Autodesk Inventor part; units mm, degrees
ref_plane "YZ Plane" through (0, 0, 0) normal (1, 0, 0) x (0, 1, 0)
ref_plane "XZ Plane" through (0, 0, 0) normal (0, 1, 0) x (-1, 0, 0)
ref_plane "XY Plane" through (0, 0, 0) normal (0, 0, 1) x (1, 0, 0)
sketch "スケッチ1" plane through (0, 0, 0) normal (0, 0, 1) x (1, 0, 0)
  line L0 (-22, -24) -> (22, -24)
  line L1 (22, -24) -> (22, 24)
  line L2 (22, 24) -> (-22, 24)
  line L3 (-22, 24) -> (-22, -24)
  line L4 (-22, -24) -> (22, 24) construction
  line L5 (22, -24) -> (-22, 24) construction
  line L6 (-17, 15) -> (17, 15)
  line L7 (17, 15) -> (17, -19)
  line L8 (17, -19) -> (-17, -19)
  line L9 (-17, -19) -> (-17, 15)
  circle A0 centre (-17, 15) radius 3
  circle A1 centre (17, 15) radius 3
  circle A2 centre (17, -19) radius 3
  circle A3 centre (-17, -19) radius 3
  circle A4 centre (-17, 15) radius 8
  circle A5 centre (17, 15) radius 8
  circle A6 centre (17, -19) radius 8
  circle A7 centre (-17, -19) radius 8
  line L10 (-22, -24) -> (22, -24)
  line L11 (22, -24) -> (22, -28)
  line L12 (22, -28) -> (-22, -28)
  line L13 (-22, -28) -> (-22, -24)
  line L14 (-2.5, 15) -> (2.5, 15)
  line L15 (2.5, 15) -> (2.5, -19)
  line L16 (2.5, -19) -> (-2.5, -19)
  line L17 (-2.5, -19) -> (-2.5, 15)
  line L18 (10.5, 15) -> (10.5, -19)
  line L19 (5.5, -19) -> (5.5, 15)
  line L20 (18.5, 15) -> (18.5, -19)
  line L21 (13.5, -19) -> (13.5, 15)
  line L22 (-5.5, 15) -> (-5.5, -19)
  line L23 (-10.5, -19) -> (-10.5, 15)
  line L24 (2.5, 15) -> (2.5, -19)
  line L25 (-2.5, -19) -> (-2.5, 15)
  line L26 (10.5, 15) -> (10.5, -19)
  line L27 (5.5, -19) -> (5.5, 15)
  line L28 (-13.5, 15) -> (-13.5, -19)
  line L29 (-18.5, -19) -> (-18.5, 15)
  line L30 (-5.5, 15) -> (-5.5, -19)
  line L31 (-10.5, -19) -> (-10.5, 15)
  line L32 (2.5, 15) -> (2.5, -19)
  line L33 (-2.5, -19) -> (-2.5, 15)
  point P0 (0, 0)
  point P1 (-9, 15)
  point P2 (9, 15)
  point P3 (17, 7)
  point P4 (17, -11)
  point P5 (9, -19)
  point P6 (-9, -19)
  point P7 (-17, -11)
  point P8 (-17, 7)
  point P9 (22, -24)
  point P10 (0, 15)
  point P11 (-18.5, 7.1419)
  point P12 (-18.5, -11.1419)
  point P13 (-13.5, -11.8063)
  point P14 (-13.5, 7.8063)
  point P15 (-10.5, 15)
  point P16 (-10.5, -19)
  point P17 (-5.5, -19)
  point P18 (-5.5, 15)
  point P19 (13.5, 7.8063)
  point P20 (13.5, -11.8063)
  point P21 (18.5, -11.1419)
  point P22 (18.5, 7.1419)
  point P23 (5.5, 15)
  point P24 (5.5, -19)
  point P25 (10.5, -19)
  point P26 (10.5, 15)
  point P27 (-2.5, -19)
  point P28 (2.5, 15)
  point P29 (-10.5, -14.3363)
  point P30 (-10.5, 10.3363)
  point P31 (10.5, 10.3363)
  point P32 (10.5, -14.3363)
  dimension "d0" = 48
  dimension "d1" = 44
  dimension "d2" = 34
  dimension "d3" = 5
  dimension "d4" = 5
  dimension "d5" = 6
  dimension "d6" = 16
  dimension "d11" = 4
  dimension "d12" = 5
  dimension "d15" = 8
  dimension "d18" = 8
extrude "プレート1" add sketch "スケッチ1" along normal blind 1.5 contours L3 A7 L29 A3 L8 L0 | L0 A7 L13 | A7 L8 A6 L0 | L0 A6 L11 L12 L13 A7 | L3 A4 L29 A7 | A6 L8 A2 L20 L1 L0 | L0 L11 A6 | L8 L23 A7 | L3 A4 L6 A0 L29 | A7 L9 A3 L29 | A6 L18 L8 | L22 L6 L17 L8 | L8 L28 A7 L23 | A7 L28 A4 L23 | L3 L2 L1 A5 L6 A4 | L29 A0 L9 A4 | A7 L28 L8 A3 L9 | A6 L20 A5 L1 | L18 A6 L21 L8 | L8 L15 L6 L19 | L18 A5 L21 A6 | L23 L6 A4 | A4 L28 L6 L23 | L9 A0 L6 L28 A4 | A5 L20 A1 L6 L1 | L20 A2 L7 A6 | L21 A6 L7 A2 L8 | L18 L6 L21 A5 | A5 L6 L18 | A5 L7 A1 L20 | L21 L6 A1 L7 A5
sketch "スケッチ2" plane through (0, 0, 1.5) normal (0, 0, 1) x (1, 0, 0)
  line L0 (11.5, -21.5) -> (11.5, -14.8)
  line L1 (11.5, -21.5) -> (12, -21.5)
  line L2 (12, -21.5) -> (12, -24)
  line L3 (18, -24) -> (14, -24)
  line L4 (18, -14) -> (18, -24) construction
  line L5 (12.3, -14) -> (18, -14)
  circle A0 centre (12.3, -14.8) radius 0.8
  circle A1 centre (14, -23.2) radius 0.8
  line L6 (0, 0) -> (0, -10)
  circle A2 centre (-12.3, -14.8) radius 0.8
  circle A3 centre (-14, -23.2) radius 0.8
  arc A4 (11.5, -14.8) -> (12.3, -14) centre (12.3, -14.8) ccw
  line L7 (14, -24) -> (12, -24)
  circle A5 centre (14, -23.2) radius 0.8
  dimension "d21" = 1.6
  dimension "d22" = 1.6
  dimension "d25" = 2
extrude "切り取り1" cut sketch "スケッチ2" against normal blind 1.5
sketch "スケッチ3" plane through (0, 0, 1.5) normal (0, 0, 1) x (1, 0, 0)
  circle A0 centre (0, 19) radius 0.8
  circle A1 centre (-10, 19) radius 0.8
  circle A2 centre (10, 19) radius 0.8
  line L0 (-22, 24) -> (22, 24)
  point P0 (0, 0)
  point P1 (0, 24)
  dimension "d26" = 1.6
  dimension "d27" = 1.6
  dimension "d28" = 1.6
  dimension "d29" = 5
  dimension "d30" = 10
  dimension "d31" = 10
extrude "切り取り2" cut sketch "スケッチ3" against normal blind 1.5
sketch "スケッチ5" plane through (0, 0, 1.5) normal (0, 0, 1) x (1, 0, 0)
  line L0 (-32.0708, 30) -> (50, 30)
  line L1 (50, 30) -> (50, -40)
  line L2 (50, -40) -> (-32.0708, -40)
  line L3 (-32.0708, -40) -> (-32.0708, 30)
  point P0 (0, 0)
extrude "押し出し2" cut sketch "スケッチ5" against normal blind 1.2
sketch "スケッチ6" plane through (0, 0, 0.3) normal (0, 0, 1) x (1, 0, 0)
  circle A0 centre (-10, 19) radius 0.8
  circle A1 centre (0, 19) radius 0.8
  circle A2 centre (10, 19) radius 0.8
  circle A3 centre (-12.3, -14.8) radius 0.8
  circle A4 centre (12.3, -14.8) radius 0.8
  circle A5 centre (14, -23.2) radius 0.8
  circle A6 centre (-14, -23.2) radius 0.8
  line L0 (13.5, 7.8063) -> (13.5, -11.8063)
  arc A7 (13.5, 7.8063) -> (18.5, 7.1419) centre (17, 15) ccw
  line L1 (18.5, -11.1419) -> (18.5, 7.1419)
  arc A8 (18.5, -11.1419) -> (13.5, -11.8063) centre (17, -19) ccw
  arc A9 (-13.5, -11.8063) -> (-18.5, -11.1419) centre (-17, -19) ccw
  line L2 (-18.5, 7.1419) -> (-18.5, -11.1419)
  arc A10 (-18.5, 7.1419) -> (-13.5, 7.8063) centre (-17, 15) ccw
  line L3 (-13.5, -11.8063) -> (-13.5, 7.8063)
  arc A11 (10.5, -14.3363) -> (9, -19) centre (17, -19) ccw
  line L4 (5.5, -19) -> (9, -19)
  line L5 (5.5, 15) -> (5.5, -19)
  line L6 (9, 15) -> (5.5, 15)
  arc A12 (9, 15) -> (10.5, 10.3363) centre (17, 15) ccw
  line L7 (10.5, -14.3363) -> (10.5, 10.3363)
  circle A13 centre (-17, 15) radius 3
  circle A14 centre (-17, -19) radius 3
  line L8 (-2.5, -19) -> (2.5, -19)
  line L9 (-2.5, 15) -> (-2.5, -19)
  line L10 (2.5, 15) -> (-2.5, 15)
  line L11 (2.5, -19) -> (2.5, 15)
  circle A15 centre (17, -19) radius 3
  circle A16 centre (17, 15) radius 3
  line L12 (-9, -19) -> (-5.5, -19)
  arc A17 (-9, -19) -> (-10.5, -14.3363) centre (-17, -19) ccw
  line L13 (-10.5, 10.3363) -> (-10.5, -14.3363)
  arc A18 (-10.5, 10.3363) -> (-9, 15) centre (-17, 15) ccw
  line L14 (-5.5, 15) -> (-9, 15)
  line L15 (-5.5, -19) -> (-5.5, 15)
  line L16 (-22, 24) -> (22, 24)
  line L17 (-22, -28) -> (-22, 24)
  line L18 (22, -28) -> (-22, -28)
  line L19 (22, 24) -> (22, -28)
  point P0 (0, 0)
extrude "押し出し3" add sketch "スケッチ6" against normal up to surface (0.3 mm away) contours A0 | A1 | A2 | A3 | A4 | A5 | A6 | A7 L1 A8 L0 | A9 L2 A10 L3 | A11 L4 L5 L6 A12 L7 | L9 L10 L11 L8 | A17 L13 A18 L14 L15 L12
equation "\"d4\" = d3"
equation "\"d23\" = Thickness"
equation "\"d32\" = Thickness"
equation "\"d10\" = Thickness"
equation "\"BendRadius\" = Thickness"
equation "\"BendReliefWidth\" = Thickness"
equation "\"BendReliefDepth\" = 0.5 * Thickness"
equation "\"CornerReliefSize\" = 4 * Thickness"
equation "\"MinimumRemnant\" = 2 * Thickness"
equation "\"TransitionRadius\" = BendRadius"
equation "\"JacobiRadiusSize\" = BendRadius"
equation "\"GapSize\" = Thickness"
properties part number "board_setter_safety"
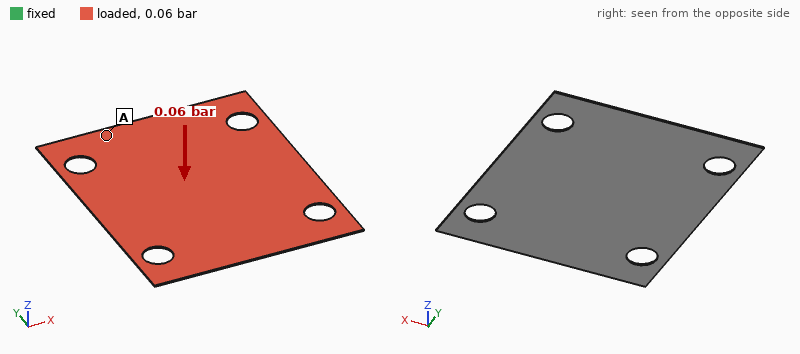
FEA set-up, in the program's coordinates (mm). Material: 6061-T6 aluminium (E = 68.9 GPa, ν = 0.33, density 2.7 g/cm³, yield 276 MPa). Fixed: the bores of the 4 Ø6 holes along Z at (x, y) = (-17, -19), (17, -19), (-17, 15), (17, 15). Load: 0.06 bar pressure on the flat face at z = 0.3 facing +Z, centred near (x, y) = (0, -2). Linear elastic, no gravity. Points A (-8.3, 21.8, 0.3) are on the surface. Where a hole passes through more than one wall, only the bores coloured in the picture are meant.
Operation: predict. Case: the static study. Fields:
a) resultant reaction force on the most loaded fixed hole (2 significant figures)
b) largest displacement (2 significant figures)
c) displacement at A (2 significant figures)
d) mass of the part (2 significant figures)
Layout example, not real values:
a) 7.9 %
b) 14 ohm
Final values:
a) 3.3 N
b) 0.18 mm
c) 0.047 mm
d) 1.8 g
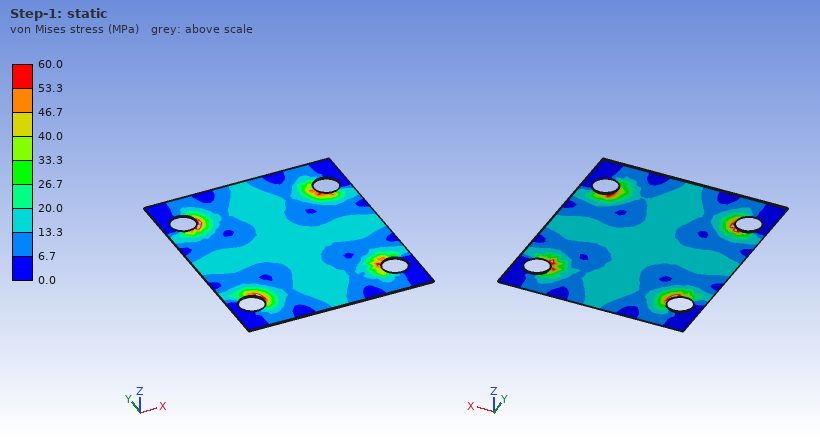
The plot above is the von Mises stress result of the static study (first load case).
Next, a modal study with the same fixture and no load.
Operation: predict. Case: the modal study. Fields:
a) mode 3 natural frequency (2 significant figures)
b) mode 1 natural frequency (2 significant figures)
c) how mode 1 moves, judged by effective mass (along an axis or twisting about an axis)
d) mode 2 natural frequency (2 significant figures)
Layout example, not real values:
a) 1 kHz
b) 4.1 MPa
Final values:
a) 1800 Hz
b) 1300 Hz
c) along Z
d) 1800 Hz
